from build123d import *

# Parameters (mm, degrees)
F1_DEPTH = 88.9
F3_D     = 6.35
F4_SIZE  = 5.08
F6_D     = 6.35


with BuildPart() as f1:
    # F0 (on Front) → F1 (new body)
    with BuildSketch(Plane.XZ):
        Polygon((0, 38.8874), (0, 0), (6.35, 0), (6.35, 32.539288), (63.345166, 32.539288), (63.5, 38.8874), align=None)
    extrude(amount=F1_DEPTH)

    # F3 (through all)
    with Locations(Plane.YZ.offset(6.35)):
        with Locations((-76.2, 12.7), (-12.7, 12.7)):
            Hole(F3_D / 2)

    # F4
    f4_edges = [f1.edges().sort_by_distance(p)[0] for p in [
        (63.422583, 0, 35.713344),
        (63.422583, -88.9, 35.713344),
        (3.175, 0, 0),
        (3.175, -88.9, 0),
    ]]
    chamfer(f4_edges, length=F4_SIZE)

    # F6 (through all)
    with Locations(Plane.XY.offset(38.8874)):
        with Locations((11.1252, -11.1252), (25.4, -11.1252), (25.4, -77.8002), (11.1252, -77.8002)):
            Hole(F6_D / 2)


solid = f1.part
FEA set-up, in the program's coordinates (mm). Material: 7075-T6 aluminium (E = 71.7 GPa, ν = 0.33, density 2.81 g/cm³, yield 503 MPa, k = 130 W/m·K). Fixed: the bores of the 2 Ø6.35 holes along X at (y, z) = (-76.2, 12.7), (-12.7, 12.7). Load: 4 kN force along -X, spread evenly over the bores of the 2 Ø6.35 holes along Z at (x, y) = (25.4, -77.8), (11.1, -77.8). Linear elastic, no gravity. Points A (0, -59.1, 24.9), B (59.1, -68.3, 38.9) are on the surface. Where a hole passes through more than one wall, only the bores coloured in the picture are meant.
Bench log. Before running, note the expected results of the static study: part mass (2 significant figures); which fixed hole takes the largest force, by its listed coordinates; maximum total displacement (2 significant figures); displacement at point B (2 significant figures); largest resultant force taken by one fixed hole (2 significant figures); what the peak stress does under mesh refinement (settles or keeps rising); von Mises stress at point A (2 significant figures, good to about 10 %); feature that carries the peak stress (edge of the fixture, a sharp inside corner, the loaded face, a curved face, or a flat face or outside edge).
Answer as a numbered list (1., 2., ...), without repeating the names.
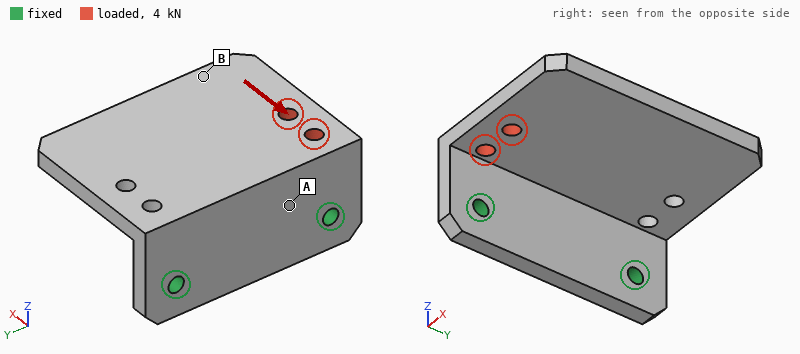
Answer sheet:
1. 150 g
2. (-76.2, 12.7)
3. 0.78 mm
4. 0.67 mm
5. 4.0 kN
6. keeps rising
7. 84 MPa
8. edge of the fixture
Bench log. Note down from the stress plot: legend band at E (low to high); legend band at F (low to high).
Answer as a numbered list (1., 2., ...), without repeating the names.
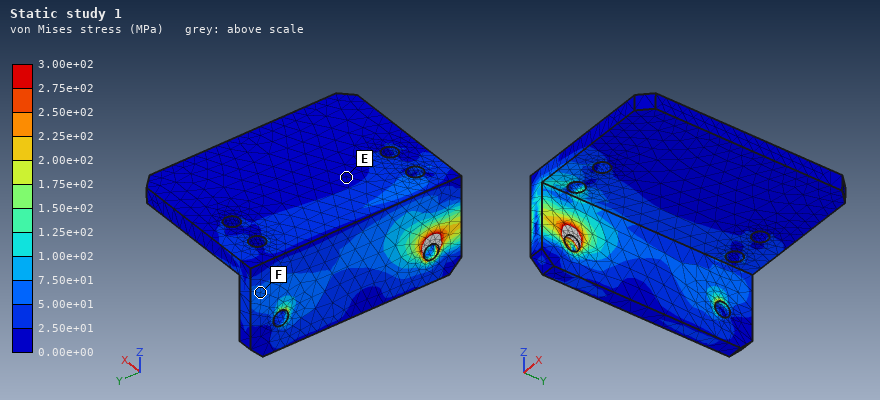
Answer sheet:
1. 0.00e+00 to 2.50e+01 MPa
2. 5.00e+01 to 7.50e+01 MPa
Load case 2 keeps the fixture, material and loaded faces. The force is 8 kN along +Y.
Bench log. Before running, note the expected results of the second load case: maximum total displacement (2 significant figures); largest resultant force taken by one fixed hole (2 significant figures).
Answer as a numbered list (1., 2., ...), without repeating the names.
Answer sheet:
1. 0.25 mm
2. 5.2 kN
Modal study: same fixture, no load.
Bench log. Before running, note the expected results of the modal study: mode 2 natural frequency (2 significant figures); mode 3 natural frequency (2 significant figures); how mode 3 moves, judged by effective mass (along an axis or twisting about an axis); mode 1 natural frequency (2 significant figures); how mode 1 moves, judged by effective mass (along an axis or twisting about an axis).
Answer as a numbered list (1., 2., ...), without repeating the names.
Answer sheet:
1. 2000 Hz
2. 2900 Hz
3. along Y
4. 870 Hz
5. along Z
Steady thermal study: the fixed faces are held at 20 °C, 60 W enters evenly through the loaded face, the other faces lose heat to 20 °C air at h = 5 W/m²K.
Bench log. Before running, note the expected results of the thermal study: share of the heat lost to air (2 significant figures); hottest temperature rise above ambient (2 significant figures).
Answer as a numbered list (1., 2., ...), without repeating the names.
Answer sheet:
1. 3.9 %
2. 59 K
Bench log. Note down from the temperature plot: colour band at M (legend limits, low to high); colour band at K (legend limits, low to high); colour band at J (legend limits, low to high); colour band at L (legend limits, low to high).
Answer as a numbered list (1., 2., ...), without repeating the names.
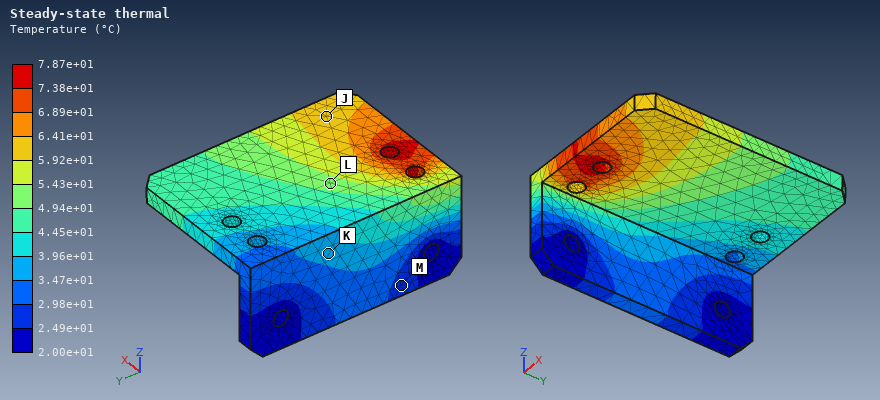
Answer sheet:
1. 2.49e+01 to 2.98e+01 °C
2. 3.47e+01 to 3.96e+01 °C
3. 5.92e+01 to 6.41e+01 °C
4. 4.94e+01 to 5.43e+01 °C
